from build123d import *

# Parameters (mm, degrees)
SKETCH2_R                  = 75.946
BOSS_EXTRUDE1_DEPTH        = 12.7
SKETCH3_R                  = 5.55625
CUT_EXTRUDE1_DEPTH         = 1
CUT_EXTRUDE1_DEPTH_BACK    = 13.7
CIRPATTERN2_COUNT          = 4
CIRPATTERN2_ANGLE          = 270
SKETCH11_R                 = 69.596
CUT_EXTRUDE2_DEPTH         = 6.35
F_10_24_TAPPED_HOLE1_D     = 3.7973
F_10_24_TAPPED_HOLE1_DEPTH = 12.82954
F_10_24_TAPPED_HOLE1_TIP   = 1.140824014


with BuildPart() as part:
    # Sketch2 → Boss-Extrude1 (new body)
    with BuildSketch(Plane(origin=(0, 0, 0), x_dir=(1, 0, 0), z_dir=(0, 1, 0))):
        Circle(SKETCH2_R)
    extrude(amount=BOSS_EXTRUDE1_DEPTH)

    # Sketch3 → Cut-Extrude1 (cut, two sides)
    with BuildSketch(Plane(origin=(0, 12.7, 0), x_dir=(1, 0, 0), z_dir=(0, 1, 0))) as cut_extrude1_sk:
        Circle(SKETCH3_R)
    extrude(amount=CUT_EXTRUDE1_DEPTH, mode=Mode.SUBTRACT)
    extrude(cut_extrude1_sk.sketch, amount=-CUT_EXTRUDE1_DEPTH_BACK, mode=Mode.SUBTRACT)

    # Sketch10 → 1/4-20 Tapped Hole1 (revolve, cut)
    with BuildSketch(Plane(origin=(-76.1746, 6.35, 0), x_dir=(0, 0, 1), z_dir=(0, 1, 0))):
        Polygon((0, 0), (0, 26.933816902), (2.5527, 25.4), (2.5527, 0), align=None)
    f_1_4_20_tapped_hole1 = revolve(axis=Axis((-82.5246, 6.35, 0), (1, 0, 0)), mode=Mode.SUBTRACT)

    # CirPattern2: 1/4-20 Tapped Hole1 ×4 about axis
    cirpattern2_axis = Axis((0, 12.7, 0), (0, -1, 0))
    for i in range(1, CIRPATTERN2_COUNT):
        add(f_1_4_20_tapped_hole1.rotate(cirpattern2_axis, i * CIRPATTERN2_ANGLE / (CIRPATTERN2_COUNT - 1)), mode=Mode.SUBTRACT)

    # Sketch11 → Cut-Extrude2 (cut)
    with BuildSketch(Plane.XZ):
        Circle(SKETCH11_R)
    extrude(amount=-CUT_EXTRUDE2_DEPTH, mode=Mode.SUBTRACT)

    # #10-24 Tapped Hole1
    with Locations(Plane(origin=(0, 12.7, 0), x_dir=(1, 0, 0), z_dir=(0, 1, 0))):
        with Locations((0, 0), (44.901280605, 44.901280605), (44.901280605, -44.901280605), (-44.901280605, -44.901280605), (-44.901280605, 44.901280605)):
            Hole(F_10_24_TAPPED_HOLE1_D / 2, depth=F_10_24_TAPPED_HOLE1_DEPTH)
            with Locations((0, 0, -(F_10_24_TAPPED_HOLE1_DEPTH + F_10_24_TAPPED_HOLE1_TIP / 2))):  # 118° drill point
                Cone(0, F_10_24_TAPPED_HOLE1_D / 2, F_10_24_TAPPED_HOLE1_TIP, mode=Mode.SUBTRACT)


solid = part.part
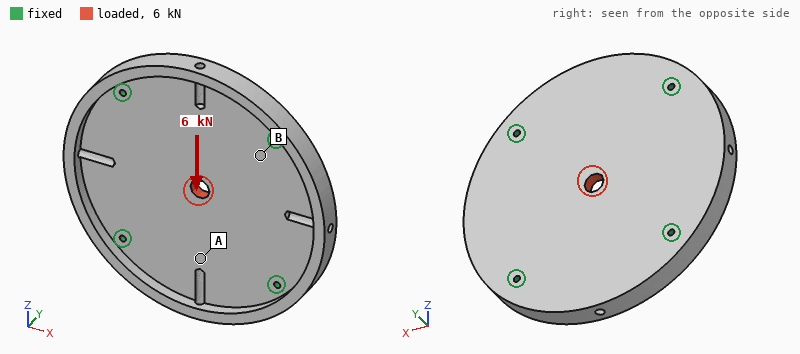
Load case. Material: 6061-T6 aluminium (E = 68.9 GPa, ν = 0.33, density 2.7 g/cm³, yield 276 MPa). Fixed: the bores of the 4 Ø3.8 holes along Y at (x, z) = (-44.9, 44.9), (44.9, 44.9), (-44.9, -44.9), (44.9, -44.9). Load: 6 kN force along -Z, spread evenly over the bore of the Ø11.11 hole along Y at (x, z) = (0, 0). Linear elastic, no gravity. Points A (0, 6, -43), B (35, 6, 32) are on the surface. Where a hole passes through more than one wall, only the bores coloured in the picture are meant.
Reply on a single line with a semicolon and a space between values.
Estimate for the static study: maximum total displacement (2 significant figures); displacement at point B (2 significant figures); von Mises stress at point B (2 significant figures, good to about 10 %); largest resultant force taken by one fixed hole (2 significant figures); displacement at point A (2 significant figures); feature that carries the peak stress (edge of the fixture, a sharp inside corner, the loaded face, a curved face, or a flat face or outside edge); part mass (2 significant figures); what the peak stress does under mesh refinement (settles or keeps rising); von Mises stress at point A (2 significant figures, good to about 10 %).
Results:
13 µm; 3.1 µm; 9.4 MPa; 1.5 kN; 6.6 µm; edge of the fixture; 350 g; keeps rising; 3.7 MPa
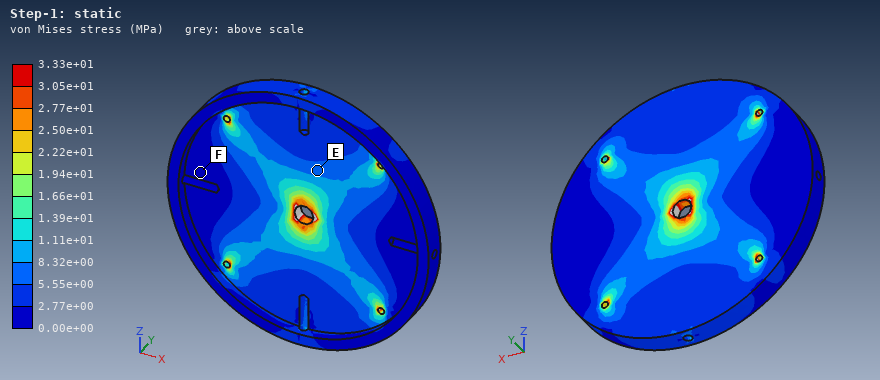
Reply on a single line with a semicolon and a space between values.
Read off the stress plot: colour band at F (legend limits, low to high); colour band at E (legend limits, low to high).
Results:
0.00e+00 to 2.77e+00 MPa; 5.55e+00 to 8.32e+00 MPa
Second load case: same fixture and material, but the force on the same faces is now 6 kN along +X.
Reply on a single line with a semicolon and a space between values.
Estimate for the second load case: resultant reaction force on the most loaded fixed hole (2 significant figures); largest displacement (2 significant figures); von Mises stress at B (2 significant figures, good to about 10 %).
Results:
1.5 kN; 13 µm; 9.2 MPa
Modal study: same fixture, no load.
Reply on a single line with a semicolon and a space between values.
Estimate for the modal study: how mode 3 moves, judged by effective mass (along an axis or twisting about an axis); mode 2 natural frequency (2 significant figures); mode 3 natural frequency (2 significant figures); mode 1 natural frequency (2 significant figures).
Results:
twisting about X; 2700 Hz; 3400 Hz; 2700 Hz
